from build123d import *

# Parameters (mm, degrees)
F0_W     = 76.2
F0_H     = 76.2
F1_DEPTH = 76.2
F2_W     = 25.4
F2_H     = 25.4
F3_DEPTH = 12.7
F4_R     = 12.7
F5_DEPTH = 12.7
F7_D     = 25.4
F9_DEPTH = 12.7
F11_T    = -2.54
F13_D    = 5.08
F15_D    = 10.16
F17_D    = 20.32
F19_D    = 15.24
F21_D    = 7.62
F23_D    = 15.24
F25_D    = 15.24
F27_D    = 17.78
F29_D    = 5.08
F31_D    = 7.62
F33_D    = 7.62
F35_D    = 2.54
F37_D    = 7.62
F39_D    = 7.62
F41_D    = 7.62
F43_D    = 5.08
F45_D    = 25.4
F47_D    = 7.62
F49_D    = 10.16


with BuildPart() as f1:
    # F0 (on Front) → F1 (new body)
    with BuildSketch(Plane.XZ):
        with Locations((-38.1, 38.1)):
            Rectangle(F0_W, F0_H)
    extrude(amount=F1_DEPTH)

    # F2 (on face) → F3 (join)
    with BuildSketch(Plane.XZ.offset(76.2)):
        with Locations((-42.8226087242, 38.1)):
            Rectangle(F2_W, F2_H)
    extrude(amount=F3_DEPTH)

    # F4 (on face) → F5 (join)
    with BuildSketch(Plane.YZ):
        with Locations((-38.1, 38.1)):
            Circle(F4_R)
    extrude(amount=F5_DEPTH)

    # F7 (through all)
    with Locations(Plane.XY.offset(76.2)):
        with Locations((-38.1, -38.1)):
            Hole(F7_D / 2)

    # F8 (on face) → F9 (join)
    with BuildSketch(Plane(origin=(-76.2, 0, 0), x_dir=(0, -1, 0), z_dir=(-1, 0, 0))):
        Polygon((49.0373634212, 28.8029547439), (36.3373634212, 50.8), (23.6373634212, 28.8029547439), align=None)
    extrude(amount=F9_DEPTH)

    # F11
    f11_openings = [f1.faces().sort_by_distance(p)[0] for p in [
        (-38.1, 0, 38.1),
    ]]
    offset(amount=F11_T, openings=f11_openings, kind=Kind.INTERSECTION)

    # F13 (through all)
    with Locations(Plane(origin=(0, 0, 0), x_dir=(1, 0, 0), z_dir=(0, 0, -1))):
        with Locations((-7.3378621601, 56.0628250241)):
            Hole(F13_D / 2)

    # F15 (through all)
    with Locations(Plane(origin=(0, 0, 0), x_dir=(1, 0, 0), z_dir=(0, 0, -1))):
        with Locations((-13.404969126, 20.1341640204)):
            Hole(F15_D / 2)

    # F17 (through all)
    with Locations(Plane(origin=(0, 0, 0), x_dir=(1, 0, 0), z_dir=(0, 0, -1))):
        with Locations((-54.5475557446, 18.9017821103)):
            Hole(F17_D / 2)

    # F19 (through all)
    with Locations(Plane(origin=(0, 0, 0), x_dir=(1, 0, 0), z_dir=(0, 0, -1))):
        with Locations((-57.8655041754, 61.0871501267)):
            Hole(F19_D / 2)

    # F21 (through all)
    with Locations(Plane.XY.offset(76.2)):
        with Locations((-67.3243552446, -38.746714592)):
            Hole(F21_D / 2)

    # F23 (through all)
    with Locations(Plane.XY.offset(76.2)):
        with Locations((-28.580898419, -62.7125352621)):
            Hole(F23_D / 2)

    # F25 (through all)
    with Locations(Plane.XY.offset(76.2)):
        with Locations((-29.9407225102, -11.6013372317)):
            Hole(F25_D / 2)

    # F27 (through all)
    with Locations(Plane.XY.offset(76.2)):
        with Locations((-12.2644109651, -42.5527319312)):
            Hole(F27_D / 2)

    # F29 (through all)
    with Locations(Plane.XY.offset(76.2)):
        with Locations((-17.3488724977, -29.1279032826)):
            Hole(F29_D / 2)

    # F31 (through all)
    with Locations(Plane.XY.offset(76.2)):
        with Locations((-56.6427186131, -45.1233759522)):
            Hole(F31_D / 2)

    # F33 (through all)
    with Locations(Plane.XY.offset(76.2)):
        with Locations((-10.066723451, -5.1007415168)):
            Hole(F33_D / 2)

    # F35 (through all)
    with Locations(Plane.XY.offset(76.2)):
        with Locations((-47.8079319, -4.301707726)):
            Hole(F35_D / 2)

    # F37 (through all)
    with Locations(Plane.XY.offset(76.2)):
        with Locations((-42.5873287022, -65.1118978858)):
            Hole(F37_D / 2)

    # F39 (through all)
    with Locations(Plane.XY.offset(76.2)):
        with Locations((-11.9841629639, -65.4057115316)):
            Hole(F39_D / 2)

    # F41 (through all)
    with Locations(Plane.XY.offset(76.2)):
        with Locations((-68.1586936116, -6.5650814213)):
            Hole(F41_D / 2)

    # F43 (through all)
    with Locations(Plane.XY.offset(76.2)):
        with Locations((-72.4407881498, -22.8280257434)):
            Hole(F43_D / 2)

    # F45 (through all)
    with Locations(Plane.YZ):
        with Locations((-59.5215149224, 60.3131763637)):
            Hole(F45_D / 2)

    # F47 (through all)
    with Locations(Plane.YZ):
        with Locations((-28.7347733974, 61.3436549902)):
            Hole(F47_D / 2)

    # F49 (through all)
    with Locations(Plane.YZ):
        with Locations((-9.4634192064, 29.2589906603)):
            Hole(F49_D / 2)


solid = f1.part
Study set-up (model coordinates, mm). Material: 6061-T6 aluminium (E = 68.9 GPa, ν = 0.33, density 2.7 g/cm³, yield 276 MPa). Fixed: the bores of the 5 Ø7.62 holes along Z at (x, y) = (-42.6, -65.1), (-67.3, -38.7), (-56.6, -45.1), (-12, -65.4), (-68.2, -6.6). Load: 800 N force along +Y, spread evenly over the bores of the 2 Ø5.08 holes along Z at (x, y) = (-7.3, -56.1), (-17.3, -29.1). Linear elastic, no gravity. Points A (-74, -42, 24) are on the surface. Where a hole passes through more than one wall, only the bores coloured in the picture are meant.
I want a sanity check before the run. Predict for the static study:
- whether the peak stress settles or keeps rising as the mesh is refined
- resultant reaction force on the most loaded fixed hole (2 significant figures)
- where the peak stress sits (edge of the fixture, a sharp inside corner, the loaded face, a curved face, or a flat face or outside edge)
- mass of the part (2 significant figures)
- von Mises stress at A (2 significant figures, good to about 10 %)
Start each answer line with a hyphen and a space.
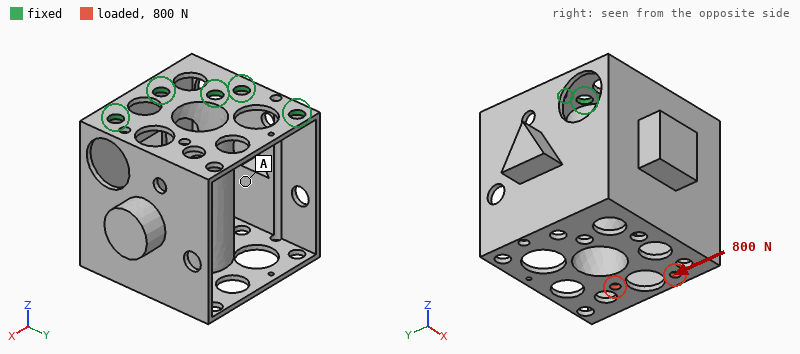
- keeps rising
- 1.1 kN
- edge of the fixture
- 210 g
- 11 MPa
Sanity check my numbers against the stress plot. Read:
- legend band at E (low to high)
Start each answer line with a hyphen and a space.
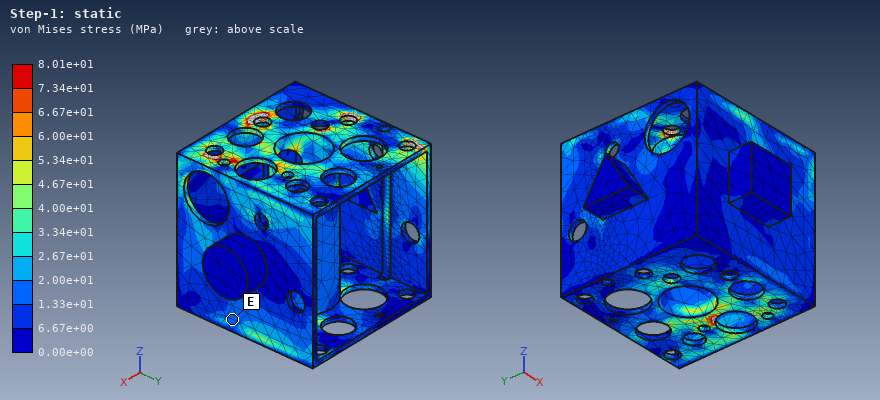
- 1.33e+01 to 2.00e+01 MPa
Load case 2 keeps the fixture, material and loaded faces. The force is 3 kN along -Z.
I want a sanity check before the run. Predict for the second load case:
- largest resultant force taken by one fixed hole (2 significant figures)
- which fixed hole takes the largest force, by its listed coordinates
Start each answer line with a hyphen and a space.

- 2.7 kN
- (-12, -65.4)
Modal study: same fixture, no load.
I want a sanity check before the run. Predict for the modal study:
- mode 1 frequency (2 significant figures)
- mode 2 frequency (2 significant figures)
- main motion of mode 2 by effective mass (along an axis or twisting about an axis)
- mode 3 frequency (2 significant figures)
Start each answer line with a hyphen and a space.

- 890 Hz
- 1100 Hz
- along X
- 1900 Hz
